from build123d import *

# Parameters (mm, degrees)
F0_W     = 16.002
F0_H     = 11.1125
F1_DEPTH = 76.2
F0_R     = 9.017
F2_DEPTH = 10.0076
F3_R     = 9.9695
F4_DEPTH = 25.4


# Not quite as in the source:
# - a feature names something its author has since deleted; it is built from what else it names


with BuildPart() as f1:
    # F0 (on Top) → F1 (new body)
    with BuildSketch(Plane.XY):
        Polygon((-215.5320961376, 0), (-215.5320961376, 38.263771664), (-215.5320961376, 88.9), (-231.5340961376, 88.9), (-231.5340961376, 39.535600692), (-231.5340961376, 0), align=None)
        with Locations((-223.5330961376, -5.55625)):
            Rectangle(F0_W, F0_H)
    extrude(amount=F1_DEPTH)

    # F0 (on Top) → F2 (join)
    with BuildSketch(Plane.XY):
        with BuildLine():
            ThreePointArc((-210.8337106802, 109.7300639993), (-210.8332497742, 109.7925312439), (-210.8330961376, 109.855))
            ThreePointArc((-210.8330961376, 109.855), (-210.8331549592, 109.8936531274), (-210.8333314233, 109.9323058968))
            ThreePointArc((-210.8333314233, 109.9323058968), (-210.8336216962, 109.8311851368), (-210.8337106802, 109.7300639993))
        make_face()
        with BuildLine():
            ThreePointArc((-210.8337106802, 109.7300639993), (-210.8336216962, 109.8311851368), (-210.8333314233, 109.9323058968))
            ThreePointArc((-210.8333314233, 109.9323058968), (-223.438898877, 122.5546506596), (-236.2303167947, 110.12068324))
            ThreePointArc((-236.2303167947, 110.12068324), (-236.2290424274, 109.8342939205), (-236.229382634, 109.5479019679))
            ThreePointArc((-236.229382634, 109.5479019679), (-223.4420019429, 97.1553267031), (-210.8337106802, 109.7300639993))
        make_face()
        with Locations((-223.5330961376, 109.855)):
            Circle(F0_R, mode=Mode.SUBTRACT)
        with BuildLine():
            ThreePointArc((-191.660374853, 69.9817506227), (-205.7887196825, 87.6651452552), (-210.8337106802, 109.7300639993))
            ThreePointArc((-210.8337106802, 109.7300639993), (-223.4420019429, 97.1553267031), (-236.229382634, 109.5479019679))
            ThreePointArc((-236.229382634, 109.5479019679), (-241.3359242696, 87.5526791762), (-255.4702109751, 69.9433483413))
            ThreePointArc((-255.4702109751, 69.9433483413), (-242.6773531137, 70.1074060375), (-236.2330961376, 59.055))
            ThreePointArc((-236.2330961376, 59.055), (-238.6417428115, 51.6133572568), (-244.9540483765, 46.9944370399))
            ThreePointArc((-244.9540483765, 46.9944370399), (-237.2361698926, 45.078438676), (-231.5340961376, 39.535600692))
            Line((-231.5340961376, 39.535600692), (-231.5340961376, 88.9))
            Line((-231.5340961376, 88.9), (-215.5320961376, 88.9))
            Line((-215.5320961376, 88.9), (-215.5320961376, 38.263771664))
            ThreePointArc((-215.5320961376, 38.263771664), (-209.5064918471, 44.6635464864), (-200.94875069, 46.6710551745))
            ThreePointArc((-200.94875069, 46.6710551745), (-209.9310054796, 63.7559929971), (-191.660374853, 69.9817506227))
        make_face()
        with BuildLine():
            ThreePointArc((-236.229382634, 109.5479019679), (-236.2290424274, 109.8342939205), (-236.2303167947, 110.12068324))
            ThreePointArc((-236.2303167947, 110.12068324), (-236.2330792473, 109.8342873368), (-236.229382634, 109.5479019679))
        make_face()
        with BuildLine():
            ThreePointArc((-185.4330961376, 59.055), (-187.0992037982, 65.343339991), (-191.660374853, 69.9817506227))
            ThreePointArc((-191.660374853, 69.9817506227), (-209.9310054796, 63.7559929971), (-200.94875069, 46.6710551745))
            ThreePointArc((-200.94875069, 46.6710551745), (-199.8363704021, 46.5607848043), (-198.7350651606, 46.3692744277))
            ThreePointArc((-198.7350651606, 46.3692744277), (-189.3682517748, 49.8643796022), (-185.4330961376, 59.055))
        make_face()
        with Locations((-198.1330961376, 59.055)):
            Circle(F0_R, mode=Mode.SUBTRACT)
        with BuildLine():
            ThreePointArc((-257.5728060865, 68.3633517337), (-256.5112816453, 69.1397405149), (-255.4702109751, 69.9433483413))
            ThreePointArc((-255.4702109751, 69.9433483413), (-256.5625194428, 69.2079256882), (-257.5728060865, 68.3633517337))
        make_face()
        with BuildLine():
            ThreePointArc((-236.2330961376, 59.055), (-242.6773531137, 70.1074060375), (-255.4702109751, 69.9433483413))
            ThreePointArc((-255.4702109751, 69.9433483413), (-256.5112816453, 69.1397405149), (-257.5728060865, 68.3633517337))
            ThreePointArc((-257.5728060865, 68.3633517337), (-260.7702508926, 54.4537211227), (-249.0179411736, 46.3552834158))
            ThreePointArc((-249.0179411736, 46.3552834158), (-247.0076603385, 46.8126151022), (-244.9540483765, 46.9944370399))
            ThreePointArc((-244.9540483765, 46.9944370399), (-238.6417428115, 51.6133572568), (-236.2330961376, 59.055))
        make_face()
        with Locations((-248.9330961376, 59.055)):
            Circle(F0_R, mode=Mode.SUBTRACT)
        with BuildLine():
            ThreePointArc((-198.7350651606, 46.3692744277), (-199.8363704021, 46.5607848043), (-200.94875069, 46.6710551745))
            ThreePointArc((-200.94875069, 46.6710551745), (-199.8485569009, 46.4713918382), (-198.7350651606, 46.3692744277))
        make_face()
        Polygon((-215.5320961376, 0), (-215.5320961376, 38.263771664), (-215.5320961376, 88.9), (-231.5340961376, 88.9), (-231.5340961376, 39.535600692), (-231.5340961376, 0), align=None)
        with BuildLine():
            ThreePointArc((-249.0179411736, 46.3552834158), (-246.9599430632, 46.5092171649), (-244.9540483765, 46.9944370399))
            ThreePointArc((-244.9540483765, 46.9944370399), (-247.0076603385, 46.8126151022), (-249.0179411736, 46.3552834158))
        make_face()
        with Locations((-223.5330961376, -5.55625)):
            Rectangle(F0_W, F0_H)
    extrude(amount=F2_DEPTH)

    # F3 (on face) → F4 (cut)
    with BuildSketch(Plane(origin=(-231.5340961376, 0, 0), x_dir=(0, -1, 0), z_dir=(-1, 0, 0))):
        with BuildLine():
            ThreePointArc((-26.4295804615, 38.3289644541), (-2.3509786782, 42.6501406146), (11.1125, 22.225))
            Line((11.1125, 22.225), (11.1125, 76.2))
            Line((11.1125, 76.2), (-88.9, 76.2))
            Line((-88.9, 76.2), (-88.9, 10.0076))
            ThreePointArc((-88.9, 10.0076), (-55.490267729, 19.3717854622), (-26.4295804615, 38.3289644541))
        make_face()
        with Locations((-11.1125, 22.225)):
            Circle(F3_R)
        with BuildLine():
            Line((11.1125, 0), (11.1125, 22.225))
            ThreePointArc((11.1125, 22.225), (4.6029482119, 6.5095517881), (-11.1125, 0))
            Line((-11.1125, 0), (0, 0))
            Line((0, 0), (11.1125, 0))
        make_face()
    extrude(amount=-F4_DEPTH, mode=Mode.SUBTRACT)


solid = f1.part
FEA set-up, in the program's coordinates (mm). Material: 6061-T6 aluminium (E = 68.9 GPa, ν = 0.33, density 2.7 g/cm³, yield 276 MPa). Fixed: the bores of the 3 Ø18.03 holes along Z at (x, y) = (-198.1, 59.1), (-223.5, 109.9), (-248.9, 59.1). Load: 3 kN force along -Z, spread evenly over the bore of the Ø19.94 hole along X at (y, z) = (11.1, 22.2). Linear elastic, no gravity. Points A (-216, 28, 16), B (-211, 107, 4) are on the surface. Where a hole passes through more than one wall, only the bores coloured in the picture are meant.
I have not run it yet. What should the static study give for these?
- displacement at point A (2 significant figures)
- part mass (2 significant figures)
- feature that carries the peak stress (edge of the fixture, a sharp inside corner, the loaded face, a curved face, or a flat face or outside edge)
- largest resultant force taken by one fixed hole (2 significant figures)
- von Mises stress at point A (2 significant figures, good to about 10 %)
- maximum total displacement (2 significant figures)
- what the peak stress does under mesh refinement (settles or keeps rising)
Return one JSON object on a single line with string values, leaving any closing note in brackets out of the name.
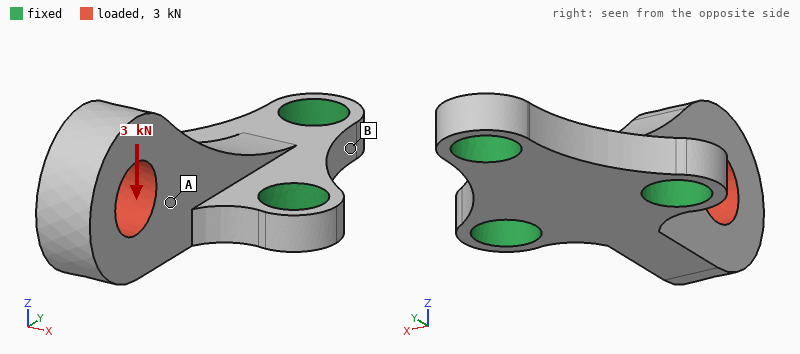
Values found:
{"displacement at point A": "0.12 mm", "part mass": "160 g", "feature that carries the peak stress": "edge of the fixture", "largest resultant force taken by one fixed hole": "2.9 kN", "von Mises stress at point A": "28 MPa", "maximum total displacement": "0.31 mm", "what the peak stress does under mesh refinement": "keeps rising"}
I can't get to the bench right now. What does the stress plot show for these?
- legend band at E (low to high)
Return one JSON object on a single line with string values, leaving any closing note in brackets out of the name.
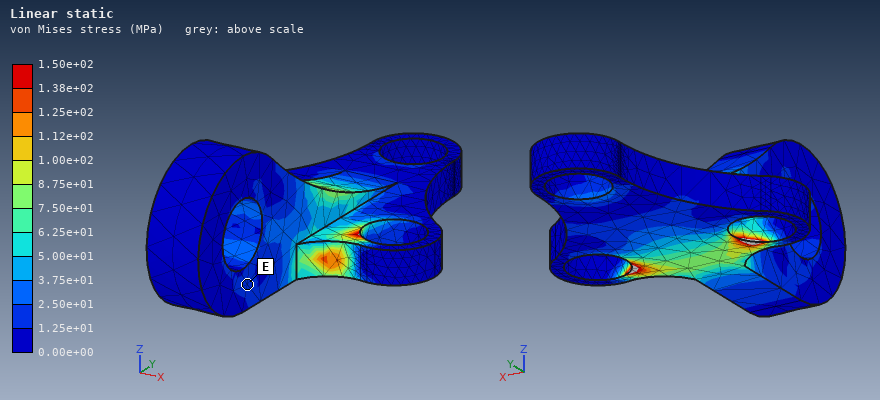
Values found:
{"legend band at E": "1.25e+01 to 2.50e+01 MPa"}
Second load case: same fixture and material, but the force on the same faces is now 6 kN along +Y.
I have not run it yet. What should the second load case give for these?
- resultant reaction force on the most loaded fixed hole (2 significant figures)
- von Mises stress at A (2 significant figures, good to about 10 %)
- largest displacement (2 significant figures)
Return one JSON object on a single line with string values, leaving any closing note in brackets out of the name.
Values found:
{"resultant reaction force on the most loaded fixed hole": "2.3 kN", "von Mises stress at A": "21 MPa", "largest displacement": "0.22 mm"}
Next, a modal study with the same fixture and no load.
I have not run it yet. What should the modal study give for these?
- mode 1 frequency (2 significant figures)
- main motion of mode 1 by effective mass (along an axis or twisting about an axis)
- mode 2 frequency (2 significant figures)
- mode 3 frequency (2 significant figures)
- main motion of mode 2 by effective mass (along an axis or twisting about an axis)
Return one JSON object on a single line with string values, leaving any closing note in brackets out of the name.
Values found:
{"mode 1 frequency": "2300 Hz", "main motion of mode 1 by effective mass": "along Z", "mode 2 frequency": "2800 Hz", "mode 3 frequency": "6400 Hz", "main motion of mode 2 by effective mass": "along X"}
